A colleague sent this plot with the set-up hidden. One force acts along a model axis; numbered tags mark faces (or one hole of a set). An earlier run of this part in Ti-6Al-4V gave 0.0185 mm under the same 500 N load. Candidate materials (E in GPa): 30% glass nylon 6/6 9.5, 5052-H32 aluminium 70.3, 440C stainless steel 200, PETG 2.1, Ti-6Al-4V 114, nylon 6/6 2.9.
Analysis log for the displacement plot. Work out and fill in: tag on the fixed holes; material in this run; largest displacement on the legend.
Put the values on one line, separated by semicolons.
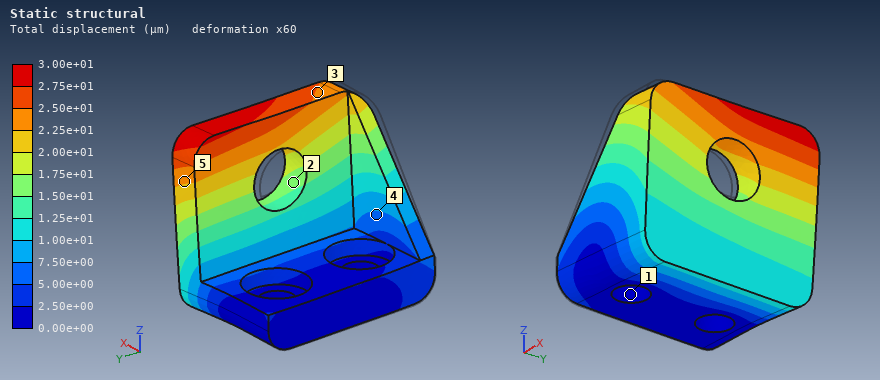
1; 5052-H32 aluminium; 3.00e+01 µm
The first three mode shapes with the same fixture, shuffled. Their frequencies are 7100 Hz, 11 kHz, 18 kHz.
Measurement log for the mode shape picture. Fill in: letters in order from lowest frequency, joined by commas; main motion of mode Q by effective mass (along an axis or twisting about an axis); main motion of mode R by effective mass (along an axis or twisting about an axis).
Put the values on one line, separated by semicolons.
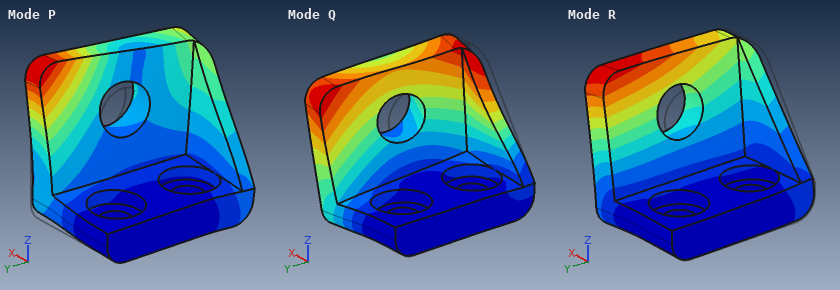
R, Q, P; along Y; along X
